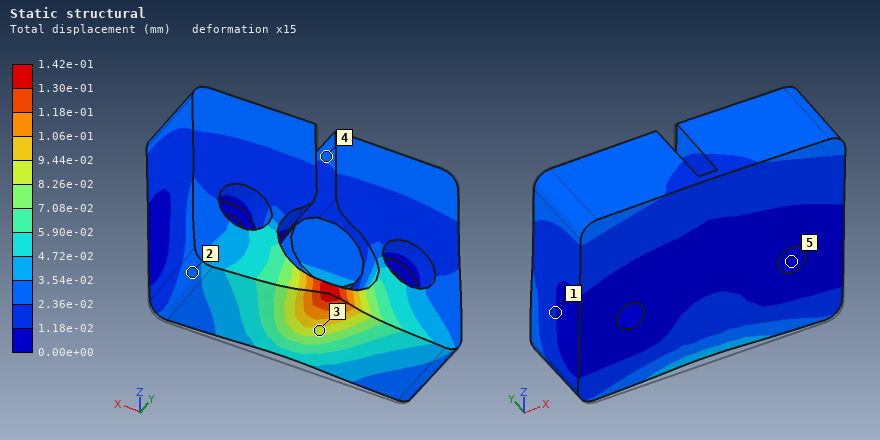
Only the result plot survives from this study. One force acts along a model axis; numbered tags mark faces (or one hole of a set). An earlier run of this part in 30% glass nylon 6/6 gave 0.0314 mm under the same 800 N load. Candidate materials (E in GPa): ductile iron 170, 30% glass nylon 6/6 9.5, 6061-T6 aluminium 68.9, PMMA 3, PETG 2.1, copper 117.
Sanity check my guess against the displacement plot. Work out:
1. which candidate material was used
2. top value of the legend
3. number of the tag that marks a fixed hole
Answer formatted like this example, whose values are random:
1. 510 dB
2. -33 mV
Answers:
1. PETG
2. 1.42e-01 mm
3. 5
